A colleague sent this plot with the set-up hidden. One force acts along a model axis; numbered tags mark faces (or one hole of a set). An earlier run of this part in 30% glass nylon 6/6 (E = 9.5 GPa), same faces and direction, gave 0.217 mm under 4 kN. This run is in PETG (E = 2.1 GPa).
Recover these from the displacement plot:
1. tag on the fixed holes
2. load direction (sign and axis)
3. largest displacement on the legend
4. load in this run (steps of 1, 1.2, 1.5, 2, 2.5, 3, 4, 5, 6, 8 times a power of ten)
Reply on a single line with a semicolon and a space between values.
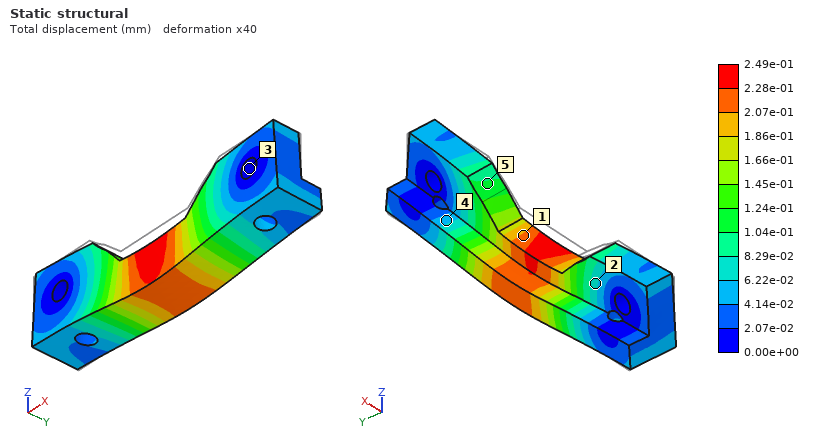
3; -Z; 2.49e-01 mm; 1 kN
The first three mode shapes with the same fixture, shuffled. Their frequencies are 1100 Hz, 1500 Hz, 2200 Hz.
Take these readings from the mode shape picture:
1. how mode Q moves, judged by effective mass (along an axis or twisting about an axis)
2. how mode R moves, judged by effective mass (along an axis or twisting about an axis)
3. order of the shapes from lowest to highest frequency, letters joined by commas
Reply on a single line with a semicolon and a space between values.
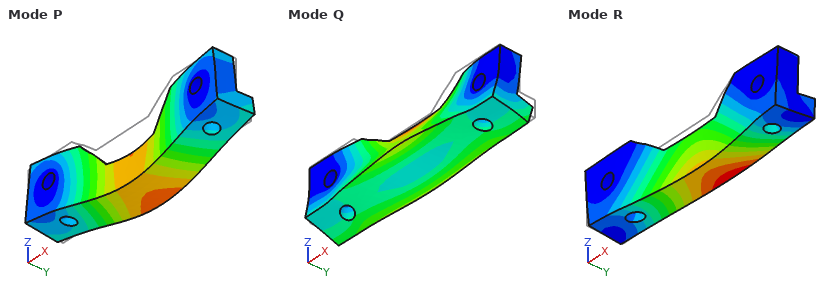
twisting about X; along Y; R, P, Q
